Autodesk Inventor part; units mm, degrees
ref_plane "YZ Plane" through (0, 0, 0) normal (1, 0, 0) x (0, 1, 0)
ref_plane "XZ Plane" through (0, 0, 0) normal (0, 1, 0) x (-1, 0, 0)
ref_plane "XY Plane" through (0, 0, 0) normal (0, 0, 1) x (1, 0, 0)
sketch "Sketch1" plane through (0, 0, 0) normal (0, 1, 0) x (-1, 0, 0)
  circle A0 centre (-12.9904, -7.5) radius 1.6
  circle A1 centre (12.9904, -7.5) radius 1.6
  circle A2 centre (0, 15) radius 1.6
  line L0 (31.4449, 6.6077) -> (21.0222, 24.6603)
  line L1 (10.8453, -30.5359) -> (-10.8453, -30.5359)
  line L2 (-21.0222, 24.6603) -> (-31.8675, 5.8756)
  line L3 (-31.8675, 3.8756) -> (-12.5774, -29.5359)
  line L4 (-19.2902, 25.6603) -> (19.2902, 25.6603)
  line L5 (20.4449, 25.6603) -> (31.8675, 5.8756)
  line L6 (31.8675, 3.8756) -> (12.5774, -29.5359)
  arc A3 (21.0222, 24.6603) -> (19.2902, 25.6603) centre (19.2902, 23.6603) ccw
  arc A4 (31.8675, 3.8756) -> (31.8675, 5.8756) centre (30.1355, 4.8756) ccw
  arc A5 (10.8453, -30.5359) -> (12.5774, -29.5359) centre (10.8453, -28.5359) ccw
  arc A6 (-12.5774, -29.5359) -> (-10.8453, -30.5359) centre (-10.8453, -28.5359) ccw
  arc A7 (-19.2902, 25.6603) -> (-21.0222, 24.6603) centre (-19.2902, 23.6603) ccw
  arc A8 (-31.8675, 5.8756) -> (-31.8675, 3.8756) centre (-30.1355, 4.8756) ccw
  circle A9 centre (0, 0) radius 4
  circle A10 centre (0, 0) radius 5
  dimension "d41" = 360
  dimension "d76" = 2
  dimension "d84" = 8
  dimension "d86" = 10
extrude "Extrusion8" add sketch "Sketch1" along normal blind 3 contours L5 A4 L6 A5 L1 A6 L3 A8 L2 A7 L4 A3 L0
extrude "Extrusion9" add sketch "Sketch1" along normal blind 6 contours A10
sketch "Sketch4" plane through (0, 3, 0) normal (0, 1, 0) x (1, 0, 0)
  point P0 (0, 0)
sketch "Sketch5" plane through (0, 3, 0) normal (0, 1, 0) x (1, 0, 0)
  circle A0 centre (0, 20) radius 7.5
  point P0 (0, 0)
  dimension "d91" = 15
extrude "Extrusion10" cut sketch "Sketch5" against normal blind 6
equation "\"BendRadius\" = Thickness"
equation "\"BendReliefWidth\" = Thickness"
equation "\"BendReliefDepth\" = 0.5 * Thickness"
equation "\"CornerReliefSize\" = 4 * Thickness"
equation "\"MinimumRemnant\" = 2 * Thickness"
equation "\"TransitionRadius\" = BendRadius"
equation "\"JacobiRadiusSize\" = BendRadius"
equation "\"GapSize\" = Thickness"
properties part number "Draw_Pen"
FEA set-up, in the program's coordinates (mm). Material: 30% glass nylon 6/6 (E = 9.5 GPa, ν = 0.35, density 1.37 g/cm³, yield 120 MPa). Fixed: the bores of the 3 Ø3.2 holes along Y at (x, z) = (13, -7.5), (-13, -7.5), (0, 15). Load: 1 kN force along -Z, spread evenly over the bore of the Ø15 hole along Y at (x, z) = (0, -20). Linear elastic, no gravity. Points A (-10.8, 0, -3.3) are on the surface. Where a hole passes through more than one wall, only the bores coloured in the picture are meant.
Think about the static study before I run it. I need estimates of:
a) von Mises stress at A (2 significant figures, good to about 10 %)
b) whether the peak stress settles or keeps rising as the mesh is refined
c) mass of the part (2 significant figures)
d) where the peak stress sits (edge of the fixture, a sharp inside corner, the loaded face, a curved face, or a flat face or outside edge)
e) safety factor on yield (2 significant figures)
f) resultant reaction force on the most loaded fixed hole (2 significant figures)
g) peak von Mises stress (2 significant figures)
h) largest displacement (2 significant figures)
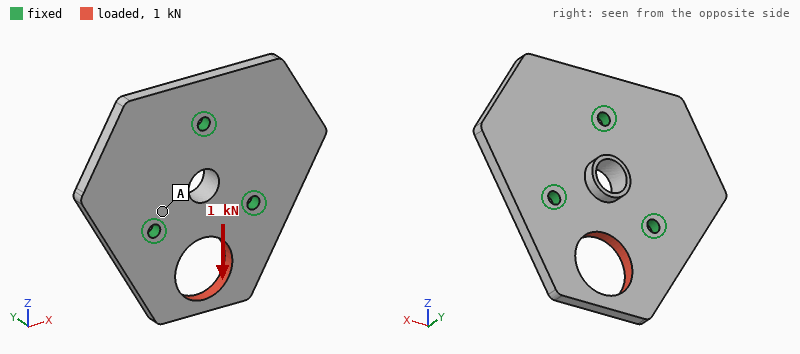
4.9 MPa
settles
10 g
a flat face or outside edge
3.1
470 N
39 MPa
67 µm
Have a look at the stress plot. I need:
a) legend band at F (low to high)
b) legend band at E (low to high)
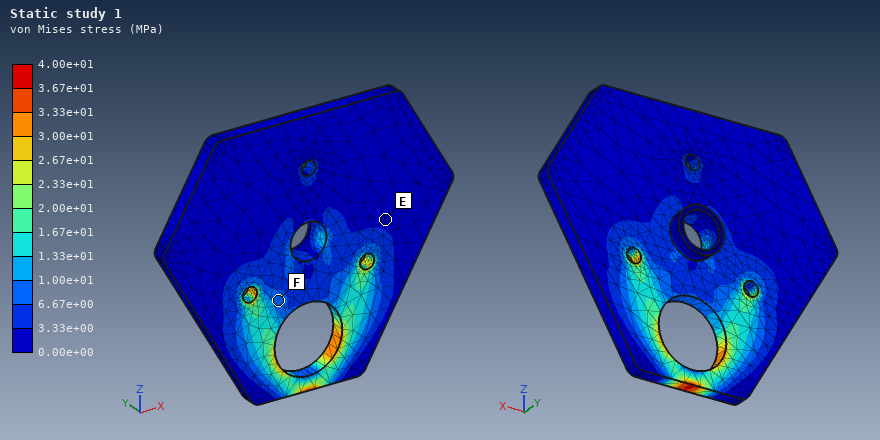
6.67e+00 to 1.00e+01 MPa
0.00e+00 to 3.33e+00 MPa
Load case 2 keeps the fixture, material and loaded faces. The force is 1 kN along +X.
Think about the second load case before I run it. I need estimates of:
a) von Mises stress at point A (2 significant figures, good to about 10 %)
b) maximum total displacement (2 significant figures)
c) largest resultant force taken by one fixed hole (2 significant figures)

4.7 MPa
0.12 mm
650 N
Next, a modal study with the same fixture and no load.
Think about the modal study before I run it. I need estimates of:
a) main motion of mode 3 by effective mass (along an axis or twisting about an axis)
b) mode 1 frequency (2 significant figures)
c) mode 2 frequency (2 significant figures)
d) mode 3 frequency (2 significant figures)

along Y
2500 Hz
2600 Hz
2900 Hz
